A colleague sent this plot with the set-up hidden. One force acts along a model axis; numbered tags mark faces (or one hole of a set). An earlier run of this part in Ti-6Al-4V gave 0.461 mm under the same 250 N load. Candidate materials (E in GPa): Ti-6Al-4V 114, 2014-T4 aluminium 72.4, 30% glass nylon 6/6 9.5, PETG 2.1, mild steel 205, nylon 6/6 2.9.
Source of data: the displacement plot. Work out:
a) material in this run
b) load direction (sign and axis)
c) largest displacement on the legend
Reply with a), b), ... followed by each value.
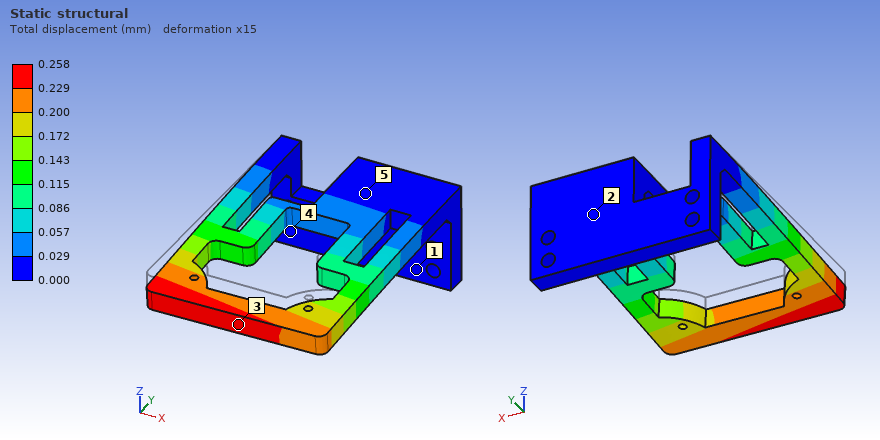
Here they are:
a) mild steel
b) -Z
c) 0.258 mm
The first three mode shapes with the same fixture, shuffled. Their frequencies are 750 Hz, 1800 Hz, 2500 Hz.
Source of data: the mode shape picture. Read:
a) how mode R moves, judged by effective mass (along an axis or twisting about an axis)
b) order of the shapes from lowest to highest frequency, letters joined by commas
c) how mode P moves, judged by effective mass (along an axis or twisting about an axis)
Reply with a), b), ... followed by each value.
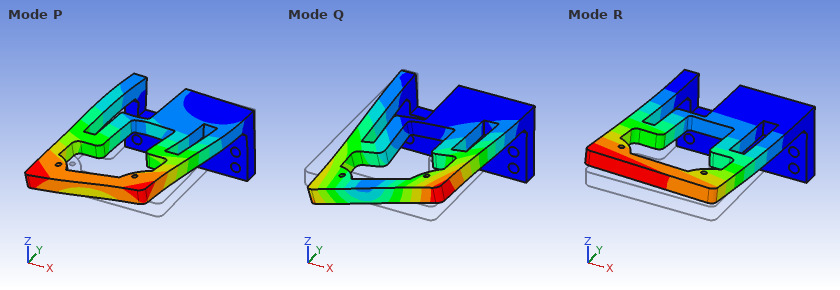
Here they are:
a) along Z
b) R, Q, P
c) along X
